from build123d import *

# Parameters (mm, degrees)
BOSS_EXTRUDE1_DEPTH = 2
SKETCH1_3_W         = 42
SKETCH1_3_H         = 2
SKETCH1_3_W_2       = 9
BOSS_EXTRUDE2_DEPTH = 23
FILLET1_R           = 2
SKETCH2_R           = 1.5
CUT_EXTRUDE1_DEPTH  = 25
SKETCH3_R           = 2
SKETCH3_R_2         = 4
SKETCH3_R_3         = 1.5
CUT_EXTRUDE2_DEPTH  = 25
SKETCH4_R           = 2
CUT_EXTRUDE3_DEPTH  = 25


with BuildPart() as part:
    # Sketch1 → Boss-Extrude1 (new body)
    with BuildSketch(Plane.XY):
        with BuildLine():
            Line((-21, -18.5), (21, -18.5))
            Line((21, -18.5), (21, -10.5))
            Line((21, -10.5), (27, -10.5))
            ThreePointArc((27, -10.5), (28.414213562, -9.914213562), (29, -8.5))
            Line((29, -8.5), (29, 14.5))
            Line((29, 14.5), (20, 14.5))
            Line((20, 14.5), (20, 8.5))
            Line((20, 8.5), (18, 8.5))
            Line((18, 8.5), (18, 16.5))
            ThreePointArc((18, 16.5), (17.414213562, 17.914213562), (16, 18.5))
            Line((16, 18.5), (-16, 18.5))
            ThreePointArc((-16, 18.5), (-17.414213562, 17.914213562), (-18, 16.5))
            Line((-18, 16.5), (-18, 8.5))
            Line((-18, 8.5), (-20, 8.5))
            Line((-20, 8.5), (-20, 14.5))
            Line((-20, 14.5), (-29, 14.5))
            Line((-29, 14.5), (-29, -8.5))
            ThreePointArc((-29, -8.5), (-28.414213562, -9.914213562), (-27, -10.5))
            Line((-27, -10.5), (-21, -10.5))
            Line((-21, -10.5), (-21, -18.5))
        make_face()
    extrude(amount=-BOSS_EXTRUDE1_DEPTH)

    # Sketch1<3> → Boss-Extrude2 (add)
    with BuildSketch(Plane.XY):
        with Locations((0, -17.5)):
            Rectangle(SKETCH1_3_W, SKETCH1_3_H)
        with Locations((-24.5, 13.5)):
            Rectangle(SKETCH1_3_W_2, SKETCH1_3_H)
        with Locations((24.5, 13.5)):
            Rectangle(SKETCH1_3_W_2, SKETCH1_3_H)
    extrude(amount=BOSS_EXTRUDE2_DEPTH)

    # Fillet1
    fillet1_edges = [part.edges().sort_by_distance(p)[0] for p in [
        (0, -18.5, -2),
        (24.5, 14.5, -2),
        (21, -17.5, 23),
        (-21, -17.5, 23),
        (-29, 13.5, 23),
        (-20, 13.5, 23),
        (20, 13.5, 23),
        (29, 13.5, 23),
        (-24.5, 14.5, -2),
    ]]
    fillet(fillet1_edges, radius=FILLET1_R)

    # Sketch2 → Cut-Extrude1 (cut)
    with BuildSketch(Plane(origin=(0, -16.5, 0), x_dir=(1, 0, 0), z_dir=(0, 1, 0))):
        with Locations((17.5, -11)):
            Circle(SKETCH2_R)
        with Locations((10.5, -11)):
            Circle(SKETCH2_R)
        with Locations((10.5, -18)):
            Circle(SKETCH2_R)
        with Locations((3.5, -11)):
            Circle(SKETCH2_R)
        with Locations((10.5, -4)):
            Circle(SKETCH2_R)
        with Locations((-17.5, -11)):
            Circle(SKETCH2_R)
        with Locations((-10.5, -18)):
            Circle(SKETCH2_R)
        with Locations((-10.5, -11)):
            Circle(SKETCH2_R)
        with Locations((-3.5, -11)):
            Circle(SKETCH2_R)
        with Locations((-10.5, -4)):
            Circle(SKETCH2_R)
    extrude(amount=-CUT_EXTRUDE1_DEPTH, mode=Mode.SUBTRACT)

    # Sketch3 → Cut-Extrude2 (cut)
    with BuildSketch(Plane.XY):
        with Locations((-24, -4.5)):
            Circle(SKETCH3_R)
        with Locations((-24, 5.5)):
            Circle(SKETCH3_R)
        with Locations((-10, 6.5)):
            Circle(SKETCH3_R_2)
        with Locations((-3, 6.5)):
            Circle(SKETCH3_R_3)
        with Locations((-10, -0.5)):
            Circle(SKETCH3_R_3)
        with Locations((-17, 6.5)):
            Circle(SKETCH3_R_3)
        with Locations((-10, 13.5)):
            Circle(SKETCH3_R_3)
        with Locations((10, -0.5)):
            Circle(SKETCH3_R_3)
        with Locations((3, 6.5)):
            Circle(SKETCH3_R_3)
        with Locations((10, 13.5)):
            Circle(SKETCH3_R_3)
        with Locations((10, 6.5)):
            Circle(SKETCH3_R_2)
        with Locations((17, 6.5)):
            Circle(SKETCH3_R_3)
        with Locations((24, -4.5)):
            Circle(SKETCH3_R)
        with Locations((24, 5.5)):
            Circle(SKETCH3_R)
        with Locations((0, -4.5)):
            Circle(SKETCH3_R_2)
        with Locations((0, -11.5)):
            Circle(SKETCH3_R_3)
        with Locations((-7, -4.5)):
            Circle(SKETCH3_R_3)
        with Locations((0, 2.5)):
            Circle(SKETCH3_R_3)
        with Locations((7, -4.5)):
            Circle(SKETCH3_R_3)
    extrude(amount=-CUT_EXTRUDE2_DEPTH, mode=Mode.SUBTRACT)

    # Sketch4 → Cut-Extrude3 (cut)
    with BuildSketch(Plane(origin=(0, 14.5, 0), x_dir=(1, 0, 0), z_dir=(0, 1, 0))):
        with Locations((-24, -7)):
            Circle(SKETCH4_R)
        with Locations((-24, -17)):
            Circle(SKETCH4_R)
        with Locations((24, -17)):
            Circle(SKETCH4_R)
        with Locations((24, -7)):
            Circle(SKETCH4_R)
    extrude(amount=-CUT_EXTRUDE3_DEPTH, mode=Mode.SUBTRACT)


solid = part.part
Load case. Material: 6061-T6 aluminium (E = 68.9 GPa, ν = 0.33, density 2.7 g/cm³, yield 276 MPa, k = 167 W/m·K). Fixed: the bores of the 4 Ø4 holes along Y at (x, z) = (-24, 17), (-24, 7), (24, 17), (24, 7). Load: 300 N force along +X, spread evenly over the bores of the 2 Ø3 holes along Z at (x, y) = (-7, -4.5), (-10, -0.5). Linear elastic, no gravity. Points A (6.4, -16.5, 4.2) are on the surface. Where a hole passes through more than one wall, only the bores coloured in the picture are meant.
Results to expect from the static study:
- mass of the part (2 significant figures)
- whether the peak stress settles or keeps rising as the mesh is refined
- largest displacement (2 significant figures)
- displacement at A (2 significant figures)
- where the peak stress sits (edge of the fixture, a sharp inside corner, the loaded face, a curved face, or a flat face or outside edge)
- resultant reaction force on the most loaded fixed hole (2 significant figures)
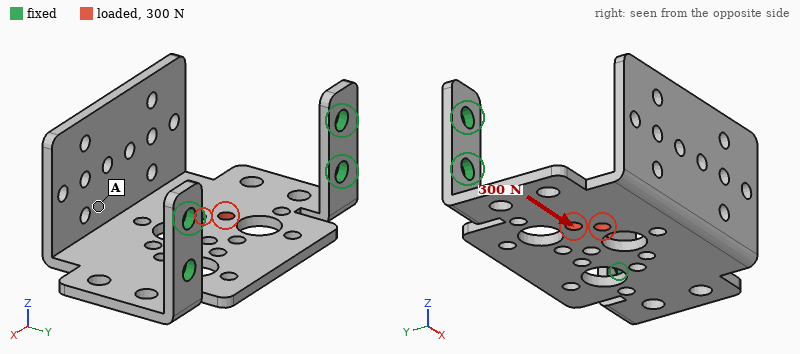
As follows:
15 g
keeps rising
90 µm
51 µm
edge of the fixture
210 N
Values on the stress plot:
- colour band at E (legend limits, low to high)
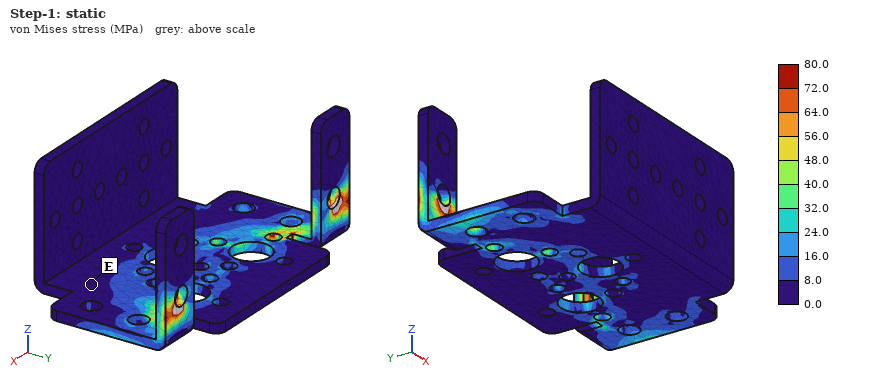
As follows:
0.0 to 8.0 MPa
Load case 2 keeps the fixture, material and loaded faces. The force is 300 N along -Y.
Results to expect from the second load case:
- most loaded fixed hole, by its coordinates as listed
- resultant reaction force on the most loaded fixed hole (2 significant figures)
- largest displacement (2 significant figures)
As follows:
(-24, 7)
210 N
0.30 mm
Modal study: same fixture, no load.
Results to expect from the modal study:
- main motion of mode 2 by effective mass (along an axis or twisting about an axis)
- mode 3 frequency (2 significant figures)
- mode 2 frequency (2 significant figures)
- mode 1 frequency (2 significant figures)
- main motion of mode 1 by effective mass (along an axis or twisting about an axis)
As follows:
along X
1600 Hz
1200 Hz
410 Hz
along Z
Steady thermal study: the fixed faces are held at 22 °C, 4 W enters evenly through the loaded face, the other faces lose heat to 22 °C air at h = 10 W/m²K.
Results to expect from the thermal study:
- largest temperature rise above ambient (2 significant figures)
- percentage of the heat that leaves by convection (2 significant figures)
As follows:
18 K
18 %
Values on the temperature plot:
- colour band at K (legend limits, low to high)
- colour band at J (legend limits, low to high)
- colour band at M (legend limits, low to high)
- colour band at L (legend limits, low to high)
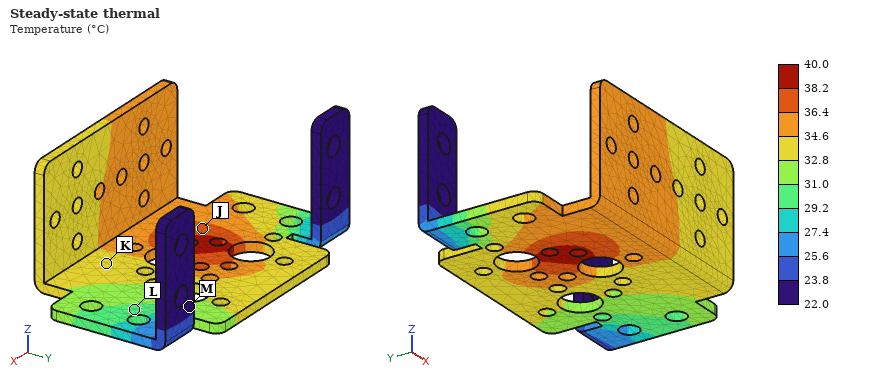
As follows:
32.8 to 34.6 °C
36.4 to 38.2 °C
22.0 to 23.8 °C
29.2 to 31.0 °C
